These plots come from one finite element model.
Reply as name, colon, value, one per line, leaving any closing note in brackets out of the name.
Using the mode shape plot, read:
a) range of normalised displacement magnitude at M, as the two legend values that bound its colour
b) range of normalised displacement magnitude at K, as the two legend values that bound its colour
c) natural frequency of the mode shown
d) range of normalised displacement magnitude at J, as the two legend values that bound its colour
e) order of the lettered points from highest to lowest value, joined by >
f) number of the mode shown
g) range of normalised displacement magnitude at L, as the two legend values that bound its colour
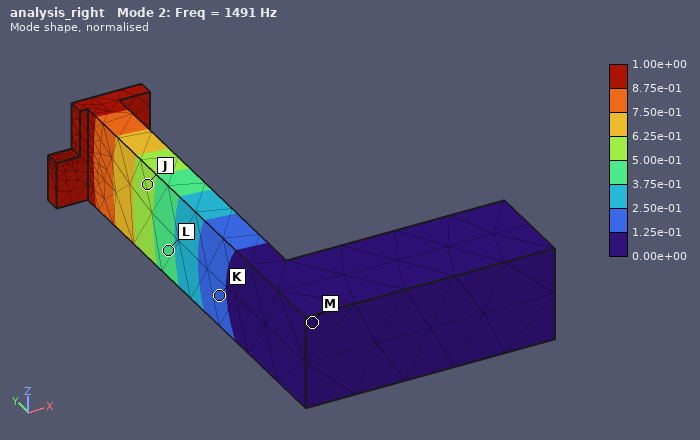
range of normalised displacement magnitude at M, as the two legend values that bound its colour: 0.00e+00 to 1.25e-01
range of normalised displacement magnitude at K, as the two legend values that bound its colour: 1.25e-01 to 2.50e-01
natural frequency of the mode shown: 1491 Hz
range of normalised displacement magnitude at J, as the two legend values that bound its colour: 5.00e-01 to 6.25e-01
order of the lettered points from highest to lowest value, joined by >: J > L > K > M
number of the mode shown: 2
range of normalised displacement magnitude at L, as the two legend values that bound its colour: 3.75e-01 to 5.00e-01
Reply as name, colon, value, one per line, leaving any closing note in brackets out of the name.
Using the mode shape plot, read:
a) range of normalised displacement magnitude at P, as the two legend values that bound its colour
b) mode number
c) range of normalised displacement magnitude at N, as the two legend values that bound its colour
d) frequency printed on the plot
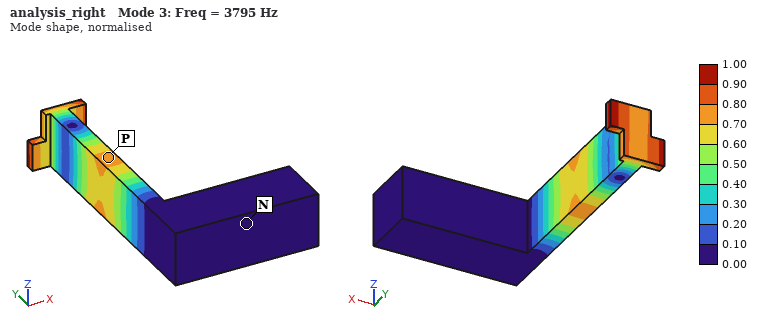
range of normalised displacement magnitude at P, as the two legend values that bound its colour: 0.70 to 0.80
mode number: 3
range of normalised displacement magnitude at N, as the two legend values that bound its colour: 0.00 to 0.10
frequency printed on the plot: 3795 Hz
